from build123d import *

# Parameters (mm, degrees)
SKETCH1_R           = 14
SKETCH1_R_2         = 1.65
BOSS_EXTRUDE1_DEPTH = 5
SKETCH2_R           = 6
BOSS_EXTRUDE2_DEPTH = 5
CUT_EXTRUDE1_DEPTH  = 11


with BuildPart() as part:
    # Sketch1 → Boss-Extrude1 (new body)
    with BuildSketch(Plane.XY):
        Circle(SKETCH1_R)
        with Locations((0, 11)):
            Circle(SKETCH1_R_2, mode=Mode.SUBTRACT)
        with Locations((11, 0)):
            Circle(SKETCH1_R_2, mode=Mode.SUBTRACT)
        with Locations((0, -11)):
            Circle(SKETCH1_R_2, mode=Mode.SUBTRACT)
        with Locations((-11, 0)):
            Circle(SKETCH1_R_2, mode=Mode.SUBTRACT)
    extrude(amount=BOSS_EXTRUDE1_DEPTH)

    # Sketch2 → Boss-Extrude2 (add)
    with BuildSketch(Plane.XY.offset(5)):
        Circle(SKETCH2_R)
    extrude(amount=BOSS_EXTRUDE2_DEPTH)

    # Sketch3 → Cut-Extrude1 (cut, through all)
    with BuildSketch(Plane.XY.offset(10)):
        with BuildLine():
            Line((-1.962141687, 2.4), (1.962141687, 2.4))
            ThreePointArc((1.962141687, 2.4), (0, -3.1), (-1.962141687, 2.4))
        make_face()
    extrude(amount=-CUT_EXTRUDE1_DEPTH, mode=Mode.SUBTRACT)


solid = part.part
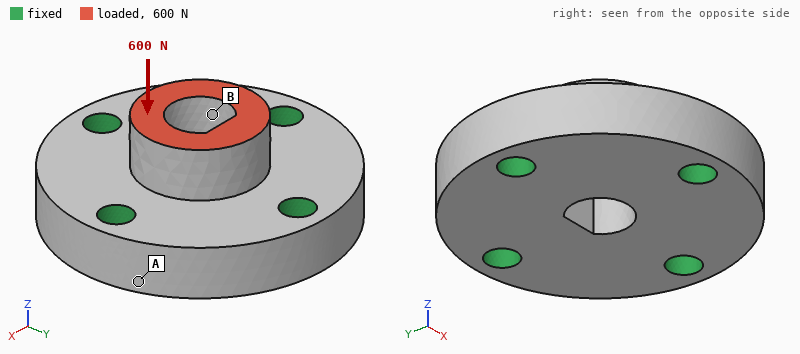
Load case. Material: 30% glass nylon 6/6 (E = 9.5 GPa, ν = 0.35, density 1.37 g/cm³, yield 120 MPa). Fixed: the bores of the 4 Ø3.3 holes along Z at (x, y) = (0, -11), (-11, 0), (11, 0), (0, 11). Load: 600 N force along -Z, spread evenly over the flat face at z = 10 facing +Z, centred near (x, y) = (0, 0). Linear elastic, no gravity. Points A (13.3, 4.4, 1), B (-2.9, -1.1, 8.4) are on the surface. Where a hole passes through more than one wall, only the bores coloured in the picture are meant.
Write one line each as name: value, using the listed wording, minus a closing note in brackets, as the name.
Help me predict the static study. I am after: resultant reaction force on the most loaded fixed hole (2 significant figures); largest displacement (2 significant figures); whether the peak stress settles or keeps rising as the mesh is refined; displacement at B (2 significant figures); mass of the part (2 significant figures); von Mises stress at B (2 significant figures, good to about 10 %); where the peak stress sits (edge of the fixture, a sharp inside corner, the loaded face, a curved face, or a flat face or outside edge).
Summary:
resultant reaction force on the most loaded fixed hole: 160 N
largest displacement: 13 µm
whether the peak stress settles or keeps rising as the mesh is refined: keeps rising
displacement at B: 11 µm
mass of the part: 4.4 g
von Mises stress at B: 5.7 MPa
where the peak stress sits: edge of the fixture
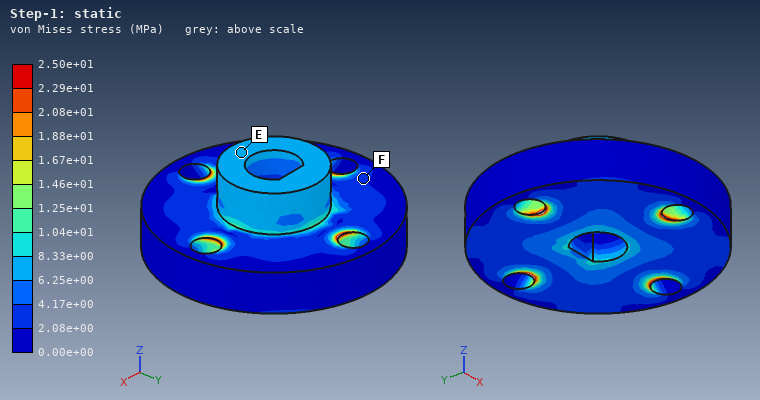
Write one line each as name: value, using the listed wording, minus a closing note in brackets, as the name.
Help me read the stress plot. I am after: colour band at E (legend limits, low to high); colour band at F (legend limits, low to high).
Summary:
colour band at E: 6.25e+00 to 8.33e+00 MPa
colour band at F: 2.08e+00 to 4.17e+00 MPa
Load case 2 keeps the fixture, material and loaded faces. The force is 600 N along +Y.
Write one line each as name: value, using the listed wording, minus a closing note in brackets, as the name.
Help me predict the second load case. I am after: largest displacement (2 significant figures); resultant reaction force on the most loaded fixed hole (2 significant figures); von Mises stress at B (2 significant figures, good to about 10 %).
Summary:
largest displacement: 45 µm
resultant reaction force on the most loaded fixed hole: 300 N
von Mises stress at B: 34 MPa
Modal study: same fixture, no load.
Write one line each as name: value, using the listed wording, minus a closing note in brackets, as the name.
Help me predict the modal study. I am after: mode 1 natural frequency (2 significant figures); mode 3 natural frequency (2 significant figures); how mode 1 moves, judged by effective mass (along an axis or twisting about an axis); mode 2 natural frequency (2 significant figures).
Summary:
mode 1 natural frequency: 31 kHz
mode 3 natural frequency: 32 kHz
how mode 1 moves, judged by effective mass: along Z
mode 2 natural frequency: 32 kHz
